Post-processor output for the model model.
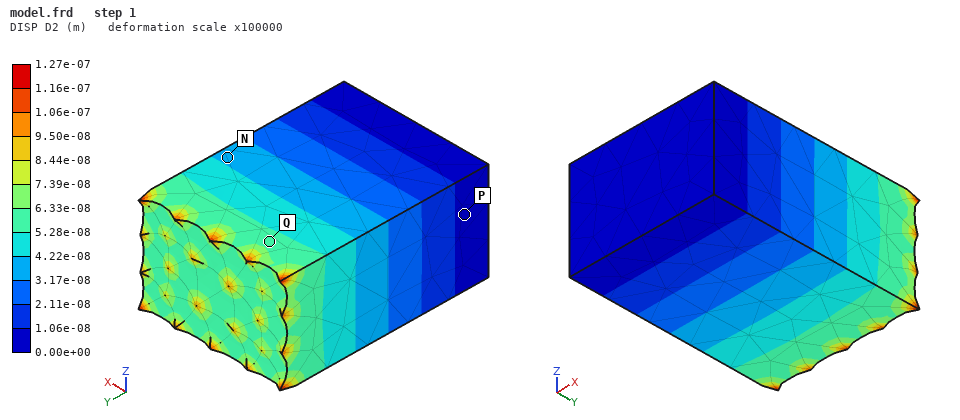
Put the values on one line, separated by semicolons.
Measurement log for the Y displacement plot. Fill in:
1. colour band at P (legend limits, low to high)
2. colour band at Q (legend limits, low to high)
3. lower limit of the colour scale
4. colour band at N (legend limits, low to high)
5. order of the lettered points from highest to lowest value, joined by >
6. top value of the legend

0.00e+00 to 1.06e-08 m; 5.28e-08 to 6.33e-08 m; 0.00e+00 m; 3.17e-08 to 4.22e-08 m; Q > N > P; 1.27e-07 m
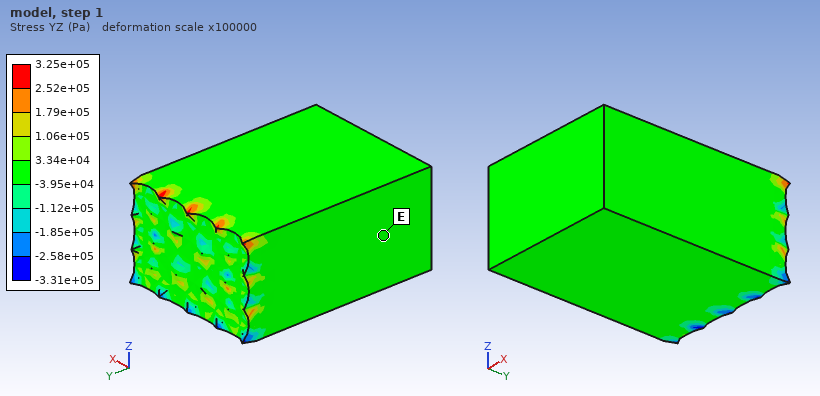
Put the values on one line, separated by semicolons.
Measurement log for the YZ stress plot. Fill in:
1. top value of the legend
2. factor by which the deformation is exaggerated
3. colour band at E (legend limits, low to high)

3.25e+05 Pa; 100000; -3.95e+04 to 3.34e+04 Pa
